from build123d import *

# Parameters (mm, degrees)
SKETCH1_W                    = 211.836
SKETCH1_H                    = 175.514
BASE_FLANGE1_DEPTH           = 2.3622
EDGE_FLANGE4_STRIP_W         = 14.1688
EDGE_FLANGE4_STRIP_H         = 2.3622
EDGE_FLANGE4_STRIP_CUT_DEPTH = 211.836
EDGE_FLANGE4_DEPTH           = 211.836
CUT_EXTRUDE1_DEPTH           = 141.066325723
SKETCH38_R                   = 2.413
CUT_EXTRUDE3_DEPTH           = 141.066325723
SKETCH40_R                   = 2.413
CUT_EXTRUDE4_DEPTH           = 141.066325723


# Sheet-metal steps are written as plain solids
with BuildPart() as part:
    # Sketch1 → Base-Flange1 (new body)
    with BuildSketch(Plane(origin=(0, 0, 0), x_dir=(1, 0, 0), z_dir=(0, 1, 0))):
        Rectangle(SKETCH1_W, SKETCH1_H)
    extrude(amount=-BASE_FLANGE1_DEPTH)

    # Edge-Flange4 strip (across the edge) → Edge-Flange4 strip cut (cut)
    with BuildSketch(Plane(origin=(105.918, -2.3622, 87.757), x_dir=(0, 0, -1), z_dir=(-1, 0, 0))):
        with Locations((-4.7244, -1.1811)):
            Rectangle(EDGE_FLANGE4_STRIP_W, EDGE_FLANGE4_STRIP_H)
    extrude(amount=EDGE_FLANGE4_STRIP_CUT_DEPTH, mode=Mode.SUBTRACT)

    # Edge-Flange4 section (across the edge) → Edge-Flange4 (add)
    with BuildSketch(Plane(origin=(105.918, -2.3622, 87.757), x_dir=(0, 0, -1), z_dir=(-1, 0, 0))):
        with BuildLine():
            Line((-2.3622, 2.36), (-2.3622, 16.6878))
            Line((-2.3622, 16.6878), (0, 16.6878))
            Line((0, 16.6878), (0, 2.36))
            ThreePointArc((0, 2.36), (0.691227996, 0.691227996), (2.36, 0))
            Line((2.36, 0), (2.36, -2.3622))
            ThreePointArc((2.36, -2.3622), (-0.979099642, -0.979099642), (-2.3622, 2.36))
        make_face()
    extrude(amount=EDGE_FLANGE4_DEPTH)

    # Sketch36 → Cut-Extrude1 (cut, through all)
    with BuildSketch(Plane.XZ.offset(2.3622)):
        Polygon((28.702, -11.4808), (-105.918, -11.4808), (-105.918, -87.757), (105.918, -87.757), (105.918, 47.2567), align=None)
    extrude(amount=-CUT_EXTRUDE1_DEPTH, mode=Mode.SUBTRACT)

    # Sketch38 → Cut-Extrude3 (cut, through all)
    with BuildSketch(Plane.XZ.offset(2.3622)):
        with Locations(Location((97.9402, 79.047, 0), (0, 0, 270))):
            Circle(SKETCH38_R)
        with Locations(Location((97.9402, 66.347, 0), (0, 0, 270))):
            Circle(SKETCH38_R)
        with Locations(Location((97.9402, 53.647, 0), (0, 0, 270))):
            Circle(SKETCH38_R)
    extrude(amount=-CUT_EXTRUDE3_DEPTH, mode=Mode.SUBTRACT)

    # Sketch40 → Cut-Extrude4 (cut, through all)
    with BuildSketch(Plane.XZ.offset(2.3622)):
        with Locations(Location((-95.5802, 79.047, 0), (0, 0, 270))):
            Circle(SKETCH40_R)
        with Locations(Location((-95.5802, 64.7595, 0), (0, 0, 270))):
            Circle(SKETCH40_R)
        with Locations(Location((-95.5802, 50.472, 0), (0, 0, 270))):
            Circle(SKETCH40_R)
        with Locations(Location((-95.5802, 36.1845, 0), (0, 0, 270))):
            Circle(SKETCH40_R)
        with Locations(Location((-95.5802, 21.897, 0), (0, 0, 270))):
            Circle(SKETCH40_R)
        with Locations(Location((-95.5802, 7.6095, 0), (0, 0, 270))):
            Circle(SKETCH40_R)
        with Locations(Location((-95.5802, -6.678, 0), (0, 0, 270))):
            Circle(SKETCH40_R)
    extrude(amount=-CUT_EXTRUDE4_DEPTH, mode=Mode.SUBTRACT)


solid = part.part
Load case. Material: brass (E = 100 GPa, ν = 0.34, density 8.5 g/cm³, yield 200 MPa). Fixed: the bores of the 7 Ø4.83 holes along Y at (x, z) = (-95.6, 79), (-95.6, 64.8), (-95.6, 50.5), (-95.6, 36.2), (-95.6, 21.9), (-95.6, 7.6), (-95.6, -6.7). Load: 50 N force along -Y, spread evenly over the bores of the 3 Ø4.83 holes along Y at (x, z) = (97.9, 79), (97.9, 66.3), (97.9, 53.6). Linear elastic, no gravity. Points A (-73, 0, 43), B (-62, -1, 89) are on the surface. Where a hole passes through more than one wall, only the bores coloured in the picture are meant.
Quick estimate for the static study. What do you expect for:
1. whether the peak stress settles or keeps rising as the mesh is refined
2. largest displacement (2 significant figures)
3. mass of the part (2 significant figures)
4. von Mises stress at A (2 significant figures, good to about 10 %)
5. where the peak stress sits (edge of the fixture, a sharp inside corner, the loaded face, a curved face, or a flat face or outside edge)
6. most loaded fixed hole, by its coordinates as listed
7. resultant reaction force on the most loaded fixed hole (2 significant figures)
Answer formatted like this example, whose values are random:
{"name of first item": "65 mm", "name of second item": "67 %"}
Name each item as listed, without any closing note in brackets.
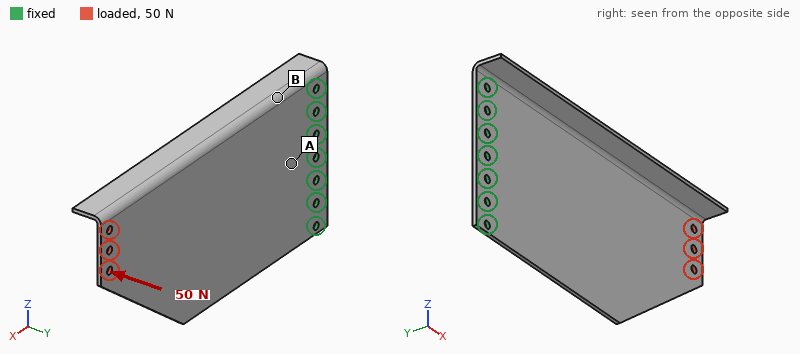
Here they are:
{"whether the peak stress settles or keeps rising as the mesh is refined": "keeps rising", "largest displacement": "2.4 mm", "mass of the part": "450 g", "von Mises stress at A": "31 MPa", "where the peak stress sits": "edge of the fixture", "most loaded fixed hole, by its coordinates as listed": "(-95.6, 79)", "resultant reaction force on the most loaded fixed hole": "220 N"}
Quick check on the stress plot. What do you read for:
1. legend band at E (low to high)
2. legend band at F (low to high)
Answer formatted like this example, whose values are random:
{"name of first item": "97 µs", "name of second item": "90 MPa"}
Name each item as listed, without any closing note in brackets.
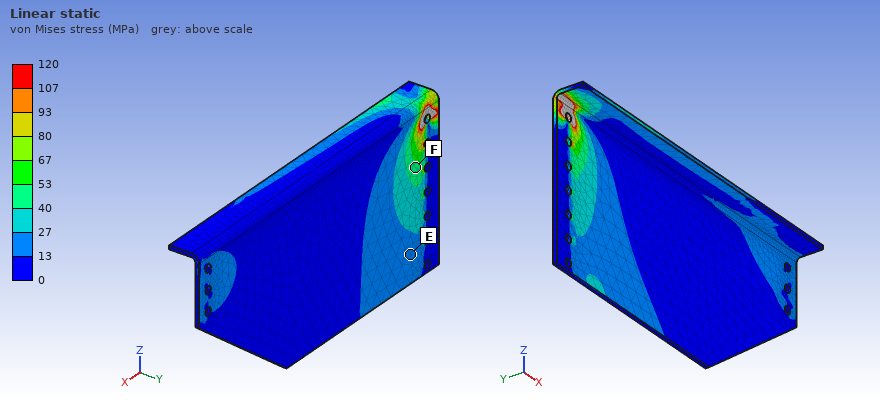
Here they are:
{"legend band at E": "13 to 27 MPa", "legend band at F": "40 to 53 MPa"}
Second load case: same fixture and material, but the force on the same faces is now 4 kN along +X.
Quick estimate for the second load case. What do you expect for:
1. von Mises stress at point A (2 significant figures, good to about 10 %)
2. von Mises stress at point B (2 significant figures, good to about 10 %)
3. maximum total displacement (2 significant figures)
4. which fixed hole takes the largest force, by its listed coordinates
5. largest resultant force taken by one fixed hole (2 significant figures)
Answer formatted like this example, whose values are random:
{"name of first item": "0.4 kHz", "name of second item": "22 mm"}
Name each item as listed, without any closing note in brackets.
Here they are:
{"von Mises stress at point A": "20 MPa", "von Mises stress at point B": "36 MPa", "maximum total displacement": "0.55 mm", "which fixed hole takes the largest force, by its listed coordinates": "(-95.6, 79)", "largest resultant force taken by one fixed hole": "1.8 kN"}
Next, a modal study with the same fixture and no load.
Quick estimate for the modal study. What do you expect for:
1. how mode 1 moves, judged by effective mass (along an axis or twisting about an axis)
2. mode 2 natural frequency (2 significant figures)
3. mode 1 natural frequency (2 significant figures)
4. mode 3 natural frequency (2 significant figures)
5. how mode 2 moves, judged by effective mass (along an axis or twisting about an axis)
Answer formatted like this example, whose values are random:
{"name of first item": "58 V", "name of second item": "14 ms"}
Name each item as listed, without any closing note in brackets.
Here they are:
{"how mode 1 moves, judged by effective mass": "along Y", "mode 2 natural frequency": "160 Hz", "mode 1 natural frequency": "71 Hz", "mode 3 natural frequency": "410 Hz", "how mode 2 moves, judged by effective mass": "twisting about X"}
